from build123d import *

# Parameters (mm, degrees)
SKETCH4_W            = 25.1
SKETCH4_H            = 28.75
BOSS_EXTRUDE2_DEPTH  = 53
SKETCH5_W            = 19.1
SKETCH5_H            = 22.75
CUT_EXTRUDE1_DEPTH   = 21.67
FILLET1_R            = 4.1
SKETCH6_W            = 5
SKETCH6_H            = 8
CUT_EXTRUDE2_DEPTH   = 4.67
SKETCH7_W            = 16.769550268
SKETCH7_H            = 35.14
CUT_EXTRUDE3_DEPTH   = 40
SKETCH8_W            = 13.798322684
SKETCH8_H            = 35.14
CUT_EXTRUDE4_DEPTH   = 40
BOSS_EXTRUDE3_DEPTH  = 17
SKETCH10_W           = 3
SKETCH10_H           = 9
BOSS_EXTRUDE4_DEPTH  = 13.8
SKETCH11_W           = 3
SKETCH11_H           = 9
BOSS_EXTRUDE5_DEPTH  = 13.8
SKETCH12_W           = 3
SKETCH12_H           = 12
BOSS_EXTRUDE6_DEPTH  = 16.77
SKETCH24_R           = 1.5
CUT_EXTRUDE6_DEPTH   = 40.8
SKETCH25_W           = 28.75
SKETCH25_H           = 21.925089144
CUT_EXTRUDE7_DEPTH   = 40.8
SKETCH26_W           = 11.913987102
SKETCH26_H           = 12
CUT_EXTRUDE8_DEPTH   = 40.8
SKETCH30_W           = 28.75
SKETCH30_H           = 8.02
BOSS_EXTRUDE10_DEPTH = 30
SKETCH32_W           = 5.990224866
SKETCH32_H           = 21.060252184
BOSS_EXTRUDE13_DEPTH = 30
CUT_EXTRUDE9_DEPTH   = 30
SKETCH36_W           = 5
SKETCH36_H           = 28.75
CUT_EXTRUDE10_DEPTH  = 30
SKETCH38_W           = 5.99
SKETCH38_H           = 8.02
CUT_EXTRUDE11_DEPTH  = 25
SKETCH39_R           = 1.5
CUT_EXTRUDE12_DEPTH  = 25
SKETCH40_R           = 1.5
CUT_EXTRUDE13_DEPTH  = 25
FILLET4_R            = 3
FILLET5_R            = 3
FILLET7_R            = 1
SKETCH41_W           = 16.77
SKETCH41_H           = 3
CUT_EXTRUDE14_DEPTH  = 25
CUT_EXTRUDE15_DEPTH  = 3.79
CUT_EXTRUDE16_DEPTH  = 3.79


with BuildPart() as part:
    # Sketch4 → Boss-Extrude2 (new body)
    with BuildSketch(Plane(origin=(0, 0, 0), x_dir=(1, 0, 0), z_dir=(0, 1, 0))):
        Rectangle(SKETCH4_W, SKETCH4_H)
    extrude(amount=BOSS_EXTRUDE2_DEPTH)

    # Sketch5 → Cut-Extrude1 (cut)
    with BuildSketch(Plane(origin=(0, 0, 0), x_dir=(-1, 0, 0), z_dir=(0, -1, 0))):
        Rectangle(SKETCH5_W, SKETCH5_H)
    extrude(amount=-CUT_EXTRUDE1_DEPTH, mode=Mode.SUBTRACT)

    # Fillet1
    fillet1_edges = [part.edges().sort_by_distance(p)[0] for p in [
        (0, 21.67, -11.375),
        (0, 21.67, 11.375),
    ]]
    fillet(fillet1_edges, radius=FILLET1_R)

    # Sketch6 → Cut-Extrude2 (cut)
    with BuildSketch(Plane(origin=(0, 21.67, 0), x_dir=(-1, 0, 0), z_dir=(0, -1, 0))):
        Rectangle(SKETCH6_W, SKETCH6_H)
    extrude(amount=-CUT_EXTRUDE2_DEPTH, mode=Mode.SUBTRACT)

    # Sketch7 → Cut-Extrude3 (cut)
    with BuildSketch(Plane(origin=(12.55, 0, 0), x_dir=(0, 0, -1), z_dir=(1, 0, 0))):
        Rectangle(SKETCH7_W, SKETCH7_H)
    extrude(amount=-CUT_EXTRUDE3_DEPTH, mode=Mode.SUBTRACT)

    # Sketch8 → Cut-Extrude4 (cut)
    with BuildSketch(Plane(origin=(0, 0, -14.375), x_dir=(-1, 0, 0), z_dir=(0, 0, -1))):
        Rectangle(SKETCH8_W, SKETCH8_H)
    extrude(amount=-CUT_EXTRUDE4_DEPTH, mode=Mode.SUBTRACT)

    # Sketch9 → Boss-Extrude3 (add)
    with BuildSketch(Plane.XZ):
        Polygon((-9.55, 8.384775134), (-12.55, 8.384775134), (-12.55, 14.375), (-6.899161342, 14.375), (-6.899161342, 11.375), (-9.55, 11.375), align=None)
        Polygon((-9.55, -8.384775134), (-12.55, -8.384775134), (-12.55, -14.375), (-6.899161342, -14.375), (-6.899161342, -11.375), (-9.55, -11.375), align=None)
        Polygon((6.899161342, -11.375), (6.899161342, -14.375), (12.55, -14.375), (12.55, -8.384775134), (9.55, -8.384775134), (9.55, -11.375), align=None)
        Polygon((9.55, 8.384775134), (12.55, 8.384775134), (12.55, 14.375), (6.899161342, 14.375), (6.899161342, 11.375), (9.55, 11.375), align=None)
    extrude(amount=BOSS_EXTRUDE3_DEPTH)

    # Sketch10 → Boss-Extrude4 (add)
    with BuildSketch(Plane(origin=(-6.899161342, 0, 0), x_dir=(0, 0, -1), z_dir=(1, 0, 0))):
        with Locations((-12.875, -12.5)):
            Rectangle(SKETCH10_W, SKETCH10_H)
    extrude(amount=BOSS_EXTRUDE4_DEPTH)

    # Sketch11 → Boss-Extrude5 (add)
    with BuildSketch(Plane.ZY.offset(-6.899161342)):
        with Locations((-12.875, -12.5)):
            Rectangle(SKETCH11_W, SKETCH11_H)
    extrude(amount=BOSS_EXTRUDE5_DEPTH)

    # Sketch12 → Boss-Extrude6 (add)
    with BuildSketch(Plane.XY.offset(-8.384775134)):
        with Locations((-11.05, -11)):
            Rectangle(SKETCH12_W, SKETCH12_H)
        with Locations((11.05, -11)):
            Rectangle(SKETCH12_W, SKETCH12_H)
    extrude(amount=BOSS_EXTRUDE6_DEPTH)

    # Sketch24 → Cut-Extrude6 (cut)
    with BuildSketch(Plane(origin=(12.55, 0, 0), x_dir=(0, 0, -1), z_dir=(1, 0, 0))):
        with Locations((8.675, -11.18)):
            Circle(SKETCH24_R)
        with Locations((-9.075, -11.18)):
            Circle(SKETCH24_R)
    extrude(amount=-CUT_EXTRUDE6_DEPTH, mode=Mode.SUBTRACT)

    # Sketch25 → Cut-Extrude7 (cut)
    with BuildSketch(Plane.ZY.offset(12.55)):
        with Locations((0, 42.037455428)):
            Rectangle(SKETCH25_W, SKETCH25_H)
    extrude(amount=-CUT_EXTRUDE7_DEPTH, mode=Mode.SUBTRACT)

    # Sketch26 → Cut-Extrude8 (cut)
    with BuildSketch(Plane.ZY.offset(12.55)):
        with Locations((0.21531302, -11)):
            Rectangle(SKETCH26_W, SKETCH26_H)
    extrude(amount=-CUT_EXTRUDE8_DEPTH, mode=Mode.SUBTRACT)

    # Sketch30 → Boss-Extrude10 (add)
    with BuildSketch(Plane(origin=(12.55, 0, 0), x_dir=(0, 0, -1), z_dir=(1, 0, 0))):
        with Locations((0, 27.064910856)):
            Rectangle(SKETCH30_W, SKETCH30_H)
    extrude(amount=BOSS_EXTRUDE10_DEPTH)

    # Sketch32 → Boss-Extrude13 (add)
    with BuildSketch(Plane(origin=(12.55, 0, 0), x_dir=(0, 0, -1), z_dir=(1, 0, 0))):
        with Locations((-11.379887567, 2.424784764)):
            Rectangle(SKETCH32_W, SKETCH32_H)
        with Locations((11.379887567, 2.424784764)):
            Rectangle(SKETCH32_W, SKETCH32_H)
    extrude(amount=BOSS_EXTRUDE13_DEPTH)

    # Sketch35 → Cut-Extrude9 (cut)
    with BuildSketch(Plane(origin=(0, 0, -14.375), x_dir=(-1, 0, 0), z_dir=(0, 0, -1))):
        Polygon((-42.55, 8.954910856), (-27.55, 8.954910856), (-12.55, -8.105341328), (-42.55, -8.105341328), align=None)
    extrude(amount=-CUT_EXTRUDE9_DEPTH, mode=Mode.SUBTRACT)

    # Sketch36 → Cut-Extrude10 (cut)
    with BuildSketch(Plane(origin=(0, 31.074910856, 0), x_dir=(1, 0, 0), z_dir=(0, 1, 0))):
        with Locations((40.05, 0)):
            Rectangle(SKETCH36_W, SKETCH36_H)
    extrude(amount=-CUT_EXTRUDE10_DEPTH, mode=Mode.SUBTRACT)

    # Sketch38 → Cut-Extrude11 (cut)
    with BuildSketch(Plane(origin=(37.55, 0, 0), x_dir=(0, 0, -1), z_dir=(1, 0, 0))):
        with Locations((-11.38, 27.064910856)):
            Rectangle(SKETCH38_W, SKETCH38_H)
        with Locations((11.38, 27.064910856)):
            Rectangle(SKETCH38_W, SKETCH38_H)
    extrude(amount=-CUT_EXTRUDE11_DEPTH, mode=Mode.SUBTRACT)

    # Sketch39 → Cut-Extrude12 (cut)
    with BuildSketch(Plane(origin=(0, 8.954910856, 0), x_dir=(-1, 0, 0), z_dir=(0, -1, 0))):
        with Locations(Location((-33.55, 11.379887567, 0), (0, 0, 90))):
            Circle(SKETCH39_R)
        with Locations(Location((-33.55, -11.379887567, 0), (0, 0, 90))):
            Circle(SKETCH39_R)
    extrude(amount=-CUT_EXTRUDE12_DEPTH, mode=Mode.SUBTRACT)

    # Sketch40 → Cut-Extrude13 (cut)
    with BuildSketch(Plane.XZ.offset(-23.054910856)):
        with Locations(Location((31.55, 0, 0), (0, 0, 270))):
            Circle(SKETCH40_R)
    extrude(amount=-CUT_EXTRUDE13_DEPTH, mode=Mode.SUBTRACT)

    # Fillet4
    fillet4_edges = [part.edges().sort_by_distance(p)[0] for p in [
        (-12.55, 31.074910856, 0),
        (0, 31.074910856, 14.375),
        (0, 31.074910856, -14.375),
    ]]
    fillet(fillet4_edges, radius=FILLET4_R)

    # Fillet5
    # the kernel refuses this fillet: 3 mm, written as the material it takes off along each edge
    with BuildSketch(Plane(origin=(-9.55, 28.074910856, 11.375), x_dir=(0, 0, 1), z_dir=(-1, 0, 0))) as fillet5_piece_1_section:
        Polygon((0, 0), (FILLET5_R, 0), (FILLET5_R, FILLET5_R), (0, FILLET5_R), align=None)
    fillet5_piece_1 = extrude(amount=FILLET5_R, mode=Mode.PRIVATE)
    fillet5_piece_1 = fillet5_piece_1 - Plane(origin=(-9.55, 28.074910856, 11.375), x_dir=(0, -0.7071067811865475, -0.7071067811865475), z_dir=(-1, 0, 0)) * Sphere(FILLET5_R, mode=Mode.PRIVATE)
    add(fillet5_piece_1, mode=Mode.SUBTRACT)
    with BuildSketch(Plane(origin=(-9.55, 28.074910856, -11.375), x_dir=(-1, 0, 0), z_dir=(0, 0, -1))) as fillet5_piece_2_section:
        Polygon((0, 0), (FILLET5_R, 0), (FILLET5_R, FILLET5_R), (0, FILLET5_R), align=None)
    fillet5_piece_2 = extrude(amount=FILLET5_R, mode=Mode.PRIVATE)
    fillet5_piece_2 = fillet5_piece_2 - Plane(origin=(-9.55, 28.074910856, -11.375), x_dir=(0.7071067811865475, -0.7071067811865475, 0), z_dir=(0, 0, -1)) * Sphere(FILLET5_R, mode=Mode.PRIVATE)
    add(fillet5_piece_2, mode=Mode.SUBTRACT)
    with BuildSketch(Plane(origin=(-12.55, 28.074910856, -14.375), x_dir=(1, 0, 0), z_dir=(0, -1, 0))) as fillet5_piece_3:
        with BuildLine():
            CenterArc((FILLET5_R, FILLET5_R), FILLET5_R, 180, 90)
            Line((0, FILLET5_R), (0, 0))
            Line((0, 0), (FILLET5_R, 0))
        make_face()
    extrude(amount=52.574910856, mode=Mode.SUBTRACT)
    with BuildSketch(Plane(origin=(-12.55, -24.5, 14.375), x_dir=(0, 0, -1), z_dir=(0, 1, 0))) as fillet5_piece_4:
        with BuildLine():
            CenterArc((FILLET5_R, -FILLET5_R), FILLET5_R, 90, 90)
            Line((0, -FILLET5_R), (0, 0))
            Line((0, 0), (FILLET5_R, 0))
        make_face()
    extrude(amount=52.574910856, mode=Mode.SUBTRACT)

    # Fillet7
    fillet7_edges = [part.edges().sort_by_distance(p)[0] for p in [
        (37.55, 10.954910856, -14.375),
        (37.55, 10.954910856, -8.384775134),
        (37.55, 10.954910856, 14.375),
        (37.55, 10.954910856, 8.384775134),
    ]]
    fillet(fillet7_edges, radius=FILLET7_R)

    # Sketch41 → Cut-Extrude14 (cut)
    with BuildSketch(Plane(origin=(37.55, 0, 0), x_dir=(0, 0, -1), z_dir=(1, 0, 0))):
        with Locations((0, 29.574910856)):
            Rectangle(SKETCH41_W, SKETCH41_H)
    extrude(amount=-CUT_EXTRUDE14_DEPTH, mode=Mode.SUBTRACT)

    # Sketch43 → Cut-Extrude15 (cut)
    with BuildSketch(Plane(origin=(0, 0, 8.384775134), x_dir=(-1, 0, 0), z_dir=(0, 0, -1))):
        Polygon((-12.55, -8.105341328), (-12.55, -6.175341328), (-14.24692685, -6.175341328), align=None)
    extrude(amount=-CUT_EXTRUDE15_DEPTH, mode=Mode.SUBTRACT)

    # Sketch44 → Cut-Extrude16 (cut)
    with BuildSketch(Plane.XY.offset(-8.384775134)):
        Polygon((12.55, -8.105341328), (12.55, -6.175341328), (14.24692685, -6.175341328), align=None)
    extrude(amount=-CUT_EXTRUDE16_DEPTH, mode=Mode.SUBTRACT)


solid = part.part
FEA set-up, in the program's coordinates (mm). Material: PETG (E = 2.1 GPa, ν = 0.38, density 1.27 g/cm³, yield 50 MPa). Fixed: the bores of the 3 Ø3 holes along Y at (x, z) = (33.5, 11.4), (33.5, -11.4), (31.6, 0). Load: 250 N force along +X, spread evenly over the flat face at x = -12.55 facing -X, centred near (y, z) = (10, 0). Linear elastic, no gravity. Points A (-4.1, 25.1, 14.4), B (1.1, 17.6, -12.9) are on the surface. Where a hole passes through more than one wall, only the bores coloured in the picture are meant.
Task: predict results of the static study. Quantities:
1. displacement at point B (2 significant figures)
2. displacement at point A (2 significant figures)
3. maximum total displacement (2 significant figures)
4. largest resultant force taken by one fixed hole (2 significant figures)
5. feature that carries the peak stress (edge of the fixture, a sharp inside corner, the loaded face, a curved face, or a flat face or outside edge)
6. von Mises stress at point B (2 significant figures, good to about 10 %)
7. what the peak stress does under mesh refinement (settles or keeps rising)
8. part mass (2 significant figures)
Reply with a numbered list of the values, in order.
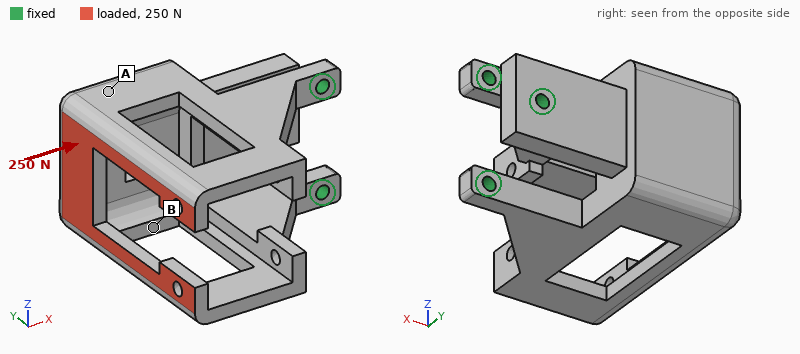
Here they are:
1. 0.23 mm
2. 0.25 mm
3. 0.78 mm
4. 110 N
5. edge of the fixture
6. 3.7 MPa
7. keeps rising
8. 21 g
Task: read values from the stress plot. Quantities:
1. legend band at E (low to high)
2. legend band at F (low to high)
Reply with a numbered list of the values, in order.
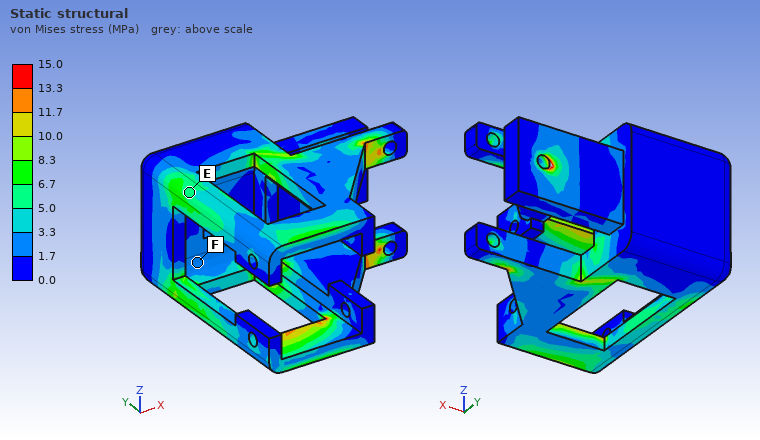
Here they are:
1. 5.0 to 6.7 MPa
2. 1.7 to 3.3 MPa
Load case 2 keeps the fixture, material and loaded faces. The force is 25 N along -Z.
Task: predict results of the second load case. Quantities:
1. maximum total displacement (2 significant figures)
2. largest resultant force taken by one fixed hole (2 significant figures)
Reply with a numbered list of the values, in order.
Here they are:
1. 0.79 mm
2. 18 N
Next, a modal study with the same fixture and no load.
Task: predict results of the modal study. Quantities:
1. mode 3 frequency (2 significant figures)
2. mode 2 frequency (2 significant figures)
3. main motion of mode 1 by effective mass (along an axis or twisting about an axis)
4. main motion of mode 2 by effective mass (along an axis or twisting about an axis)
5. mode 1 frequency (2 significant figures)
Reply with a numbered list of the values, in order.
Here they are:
1. 690 Hz
2. 620 Hz
3. along Z
4. along Y
5. 400 Hz
